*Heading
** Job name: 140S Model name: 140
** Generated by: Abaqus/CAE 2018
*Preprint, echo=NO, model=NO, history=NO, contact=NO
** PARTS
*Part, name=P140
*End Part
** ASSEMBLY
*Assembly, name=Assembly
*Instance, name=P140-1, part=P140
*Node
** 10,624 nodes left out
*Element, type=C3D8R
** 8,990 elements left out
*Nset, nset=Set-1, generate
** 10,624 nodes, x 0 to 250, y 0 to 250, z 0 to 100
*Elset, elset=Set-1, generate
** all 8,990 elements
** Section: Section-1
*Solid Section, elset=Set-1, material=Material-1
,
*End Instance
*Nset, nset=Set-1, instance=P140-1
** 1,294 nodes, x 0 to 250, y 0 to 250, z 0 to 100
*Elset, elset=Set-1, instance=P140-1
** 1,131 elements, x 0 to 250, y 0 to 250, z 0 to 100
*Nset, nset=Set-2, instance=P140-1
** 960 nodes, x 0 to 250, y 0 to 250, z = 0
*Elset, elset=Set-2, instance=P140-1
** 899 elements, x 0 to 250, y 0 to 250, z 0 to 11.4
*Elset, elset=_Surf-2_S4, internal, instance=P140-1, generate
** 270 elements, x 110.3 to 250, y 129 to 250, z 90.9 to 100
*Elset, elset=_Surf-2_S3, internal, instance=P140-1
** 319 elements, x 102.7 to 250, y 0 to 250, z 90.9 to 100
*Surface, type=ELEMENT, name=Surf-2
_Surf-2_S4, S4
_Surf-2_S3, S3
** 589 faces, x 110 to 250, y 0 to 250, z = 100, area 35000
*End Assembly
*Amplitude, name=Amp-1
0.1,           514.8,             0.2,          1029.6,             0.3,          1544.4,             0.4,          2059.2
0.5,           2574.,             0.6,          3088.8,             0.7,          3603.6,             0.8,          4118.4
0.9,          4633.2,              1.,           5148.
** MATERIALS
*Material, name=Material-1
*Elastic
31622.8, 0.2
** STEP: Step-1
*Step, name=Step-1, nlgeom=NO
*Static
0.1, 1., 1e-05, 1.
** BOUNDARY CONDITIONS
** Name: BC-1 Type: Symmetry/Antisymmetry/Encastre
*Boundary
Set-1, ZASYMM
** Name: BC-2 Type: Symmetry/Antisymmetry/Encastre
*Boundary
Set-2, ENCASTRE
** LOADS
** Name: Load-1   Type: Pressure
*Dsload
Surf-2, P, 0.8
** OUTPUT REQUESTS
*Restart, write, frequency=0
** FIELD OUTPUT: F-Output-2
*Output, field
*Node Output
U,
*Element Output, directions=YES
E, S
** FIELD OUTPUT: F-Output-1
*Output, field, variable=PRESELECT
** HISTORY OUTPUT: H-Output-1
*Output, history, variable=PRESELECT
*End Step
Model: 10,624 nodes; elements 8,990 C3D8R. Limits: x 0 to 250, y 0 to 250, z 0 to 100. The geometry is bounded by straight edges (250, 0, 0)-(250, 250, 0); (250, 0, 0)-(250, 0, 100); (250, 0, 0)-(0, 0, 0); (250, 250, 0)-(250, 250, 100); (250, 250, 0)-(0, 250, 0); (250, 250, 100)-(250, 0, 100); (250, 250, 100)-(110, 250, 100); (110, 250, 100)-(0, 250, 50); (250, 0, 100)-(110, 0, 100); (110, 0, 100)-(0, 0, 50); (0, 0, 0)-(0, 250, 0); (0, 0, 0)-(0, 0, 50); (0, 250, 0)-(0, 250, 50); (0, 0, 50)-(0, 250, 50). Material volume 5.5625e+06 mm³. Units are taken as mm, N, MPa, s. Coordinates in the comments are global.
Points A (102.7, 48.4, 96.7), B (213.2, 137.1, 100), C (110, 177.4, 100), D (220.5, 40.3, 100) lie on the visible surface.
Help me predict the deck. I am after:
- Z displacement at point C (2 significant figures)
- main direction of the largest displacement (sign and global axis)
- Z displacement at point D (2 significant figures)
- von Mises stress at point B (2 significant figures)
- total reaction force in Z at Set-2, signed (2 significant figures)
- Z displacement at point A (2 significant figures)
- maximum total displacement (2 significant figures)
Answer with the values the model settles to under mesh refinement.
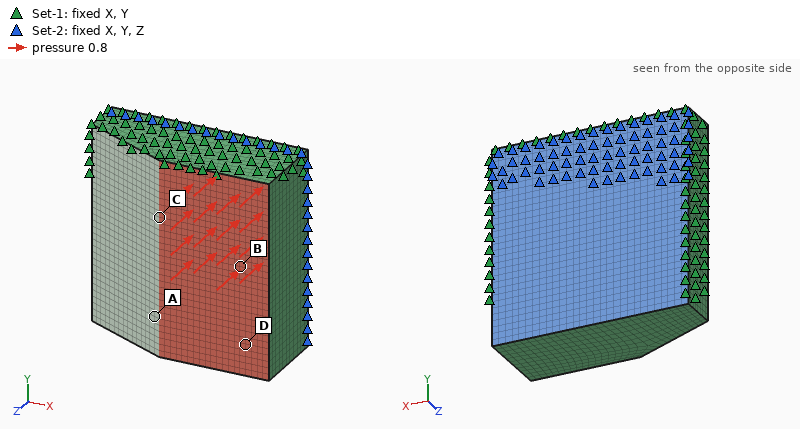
-0.0011 mm
-Z
-0.0023 mm
0.57 MPa
28000 N
-7.8e-04 mm
0.0023 mm
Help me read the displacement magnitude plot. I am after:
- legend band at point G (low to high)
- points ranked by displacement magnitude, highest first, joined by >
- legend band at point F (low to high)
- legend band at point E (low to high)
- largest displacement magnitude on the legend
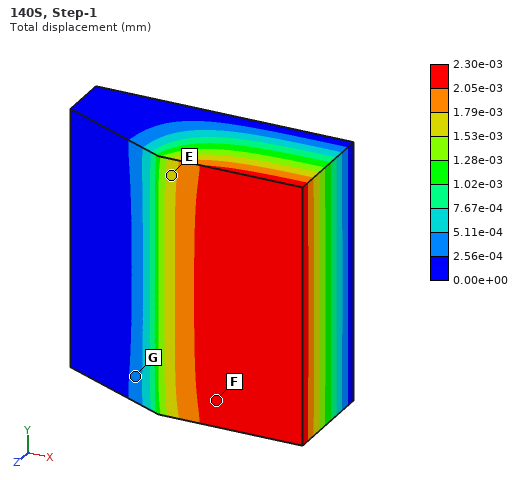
2.56e-04 to 5.11e-04 mm
F > E > G
2.05e-03 to 2.30e-03 mm
1.53e-03 to 1.79e-03 mm
2.30e-03 mm
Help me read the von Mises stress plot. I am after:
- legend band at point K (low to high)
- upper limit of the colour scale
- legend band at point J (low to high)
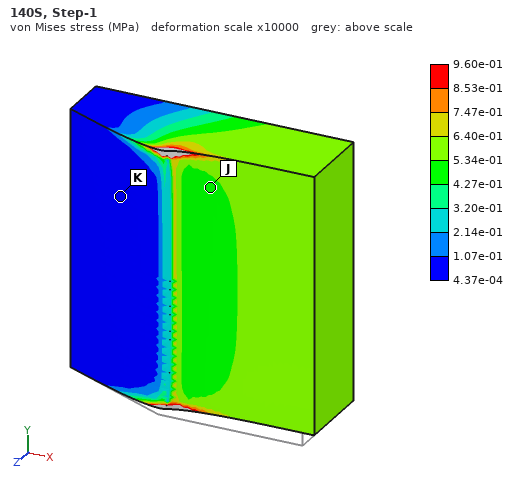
4.37e-04 to 1.07e-01 MPa
9.60e-01 MPa
4.27e-01 to 5.34e-01 MPa
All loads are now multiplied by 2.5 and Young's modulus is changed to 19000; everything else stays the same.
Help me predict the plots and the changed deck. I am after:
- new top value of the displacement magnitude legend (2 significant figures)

0.0096 mm
